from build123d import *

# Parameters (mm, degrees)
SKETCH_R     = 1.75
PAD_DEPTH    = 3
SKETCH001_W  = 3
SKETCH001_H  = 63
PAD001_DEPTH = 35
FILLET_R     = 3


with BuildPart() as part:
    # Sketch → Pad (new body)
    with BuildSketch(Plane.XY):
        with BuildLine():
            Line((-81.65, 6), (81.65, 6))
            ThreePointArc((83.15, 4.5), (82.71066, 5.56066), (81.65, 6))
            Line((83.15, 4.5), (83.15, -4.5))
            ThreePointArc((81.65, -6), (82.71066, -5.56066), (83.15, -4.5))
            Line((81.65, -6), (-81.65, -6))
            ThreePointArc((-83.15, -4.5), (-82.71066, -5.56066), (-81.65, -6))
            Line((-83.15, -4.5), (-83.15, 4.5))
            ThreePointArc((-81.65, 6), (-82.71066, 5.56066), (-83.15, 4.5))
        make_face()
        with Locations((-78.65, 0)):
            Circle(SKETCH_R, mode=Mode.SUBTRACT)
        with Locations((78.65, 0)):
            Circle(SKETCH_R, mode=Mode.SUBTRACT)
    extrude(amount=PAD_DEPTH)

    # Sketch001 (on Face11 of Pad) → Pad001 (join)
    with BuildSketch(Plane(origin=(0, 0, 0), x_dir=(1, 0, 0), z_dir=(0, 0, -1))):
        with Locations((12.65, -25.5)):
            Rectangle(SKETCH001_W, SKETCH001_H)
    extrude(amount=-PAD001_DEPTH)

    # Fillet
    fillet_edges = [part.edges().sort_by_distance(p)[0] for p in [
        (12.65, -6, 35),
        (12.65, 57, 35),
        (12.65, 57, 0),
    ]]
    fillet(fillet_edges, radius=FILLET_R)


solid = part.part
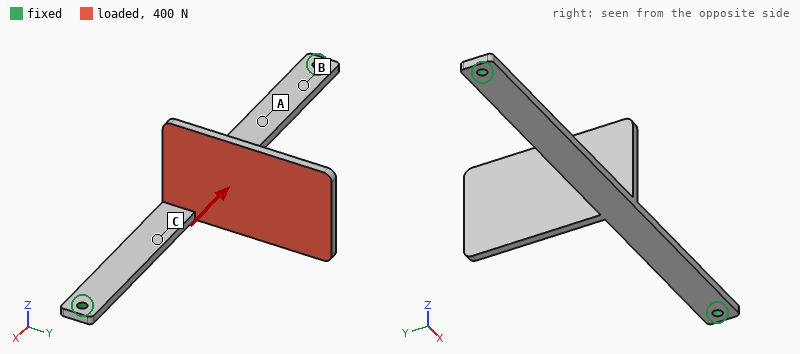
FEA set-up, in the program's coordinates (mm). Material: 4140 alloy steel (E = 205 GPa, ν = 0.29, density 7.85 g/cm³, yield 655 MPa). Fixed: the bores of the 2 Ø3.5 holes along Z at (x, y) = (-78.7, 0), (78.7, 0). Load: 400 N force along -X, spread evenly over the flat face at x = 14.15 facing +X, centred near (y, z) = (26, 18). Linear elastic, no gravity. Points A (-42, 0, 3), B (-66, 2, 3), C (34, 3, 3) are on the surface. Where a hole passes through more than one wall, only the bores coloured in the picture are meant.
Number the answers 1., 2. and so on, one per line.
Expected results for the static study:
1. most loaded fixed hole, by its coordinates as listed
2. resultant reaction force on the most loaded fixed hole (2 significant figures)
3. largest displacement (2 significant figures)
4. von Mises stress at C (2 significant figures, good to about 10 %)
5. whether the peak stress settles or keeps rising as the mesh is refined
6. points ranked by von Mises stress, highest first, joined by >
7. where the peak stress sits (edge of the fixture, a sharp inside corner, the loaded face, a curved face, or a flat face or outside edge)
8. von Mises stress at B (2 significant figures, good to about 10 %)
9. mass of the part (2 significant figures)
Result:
1. (78.7, 0)
2. 250 N
3. 1.4 mm
4. 120 MPa
5. keeps rising
6. C > B > A
7. a sharp inside corner
8. 72 MPa
9. 97 g
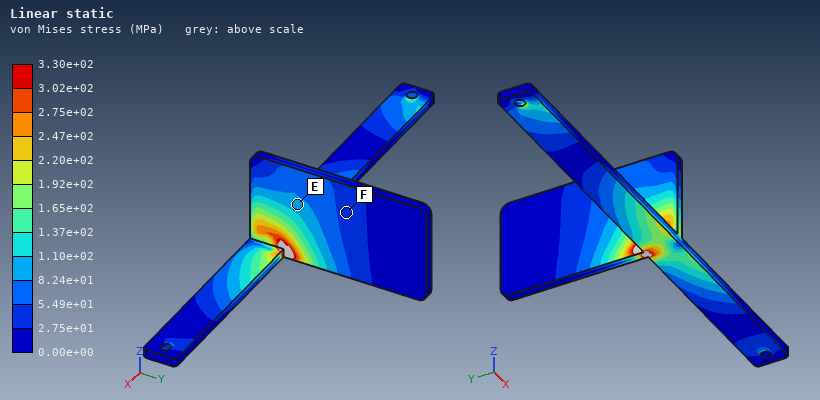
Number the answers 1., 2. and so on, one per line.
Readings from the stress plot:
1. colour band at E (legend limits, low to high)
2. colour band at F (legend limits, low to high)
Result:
1. 8.24e+01 to 1.10e+02 MPa
2. 2.75e+01 to 5.49e+01 MPa
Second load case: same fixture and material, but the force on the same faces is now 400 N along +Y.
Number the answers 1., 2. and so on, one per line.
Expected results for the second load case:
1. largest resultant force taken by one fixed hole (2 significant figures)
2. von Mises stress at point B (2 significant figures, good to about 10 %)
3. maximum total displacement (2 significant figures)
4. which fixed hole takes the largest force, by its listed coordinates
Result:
1. 250 N
2. 160 MPa
3. 2.2 mm
4. (78.7, 0)
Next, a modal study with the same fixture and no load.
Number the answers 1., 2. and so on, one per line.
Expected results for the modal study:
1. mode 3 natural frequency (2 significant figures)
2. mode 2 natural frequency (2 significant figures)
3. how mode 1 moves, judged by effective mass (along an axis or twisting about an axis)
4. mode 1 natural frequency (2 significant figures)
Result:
1. 540 Hz
2. 460 Hz
3. along Z
4. 230 Hz
